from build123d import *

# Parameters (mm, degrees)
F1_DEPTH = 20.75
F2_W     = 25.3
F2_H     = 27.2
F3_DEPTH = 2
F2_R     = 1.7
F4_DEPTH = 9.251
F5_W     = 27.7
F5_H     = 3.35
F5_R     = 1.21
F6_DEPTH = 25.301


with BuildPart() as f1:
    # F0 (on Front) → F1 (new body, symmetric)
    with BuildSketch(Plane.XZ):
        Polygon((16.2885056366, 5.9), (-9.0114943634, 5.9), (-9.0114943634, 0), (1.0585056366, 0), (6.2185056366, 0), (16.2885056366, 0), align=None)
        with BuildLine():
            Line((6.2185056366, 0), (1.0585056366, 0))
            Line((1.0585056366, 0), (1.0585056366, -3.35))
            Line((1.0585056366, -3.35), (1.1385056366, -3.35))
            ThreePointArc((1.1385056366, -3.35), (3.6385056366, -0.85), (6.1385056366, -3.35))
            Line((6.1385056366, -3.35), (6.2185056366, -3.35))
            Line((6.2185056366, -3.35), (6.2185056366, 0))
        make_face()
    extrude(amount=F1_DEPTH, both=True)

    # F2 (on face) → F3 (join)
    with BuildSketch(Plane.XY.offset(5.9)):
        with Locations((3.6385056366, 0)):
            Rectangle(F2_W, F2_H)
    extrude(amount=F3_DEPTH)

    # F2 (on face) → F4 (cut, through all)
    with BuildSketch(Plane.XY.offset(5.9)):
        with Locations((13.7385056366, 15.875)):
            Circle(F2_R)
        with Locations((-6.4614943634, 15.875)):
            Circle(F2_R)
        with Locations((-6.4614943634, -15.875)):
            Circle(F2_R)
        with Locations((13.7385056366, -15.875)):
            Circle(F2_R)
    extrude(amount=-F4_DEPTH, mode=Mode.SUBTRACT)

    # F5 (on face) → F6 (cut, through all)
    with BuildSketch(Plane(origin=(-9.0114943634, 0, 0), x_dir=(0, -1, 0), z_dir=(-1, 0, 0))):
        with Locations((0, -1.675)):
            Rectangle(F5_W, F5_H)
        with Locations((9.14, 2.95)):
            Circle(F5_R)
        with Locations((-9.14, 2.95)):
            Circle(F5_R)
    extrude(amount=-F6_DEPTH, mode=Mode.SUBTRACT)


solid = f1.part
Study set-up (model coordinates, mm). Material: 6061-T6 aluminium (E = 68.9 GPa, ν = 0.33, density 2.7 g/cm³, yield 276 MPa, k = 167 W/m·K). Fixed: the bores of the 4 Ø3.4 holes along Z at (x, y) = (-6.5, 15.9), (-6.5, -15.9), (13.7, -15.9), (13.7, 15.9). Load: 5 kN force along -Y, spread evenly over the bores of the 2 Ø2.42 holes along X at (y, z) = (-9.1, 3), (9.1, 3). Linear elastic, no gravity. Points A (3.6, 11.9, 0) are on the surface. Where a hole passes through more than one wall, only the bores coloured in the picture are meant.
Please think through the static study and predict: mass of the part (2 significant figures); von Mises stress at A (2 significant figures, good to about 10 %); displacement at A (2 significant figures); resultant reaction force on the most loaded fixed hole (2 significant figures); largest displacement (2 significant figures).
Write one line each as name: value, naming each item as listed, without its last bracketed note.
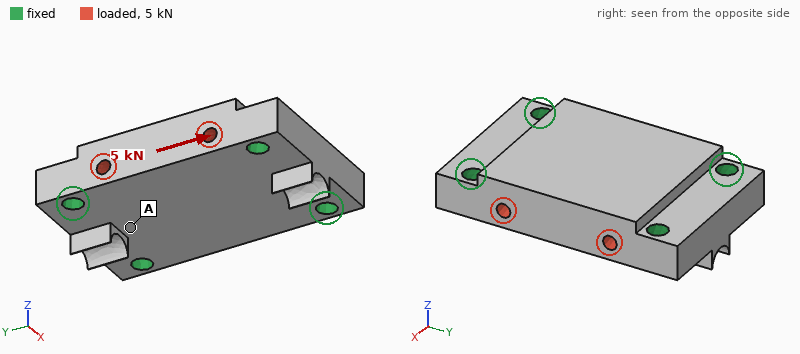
mass of the part: 20 g
von Mises stress at A: 7.4 MPa
displacement at A: 3.0 µm
resultant reaction force on the most loaded fixed hole: 1.3 kN
largest displacement: 3.5 µm
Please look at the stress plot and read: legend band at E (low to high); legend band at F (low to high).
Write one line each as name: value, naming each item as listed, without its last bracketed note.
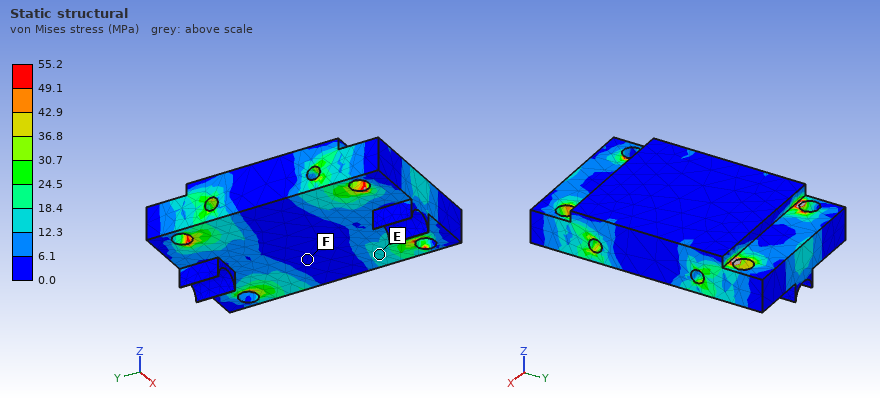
legend band at E: 12.3 to 18.4 MPa
legend band at F: 0.0 to 6.1 MPa
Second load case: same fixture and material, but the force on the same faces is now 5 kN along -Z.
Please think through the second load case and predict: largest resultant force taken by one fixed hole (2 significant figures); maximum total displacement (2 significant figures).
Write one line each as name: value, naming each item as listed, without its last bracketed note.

largest resultant force taken by one fixed hole: 1.3 kN
maximum total displacement: 15 µm
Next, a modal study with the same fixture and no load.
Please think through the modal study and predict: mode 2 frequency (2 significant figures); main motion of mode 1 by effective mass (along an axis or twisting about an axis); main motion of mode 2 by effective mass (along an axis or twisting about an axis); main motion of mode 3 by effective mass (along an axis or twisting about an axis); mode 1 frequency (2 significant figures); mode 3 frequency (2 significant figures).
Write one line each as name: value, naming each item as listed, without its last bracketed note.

mode 2 frequency: 33 kHz
main motion of mode 1 by effective mass: along Z
main motion of mode 2 by effective mass: twisting about Y
main motion of mode 3 by effective mass: along X
mode 1 frequency: 24 kHz
mode 3 frequency: 39 kHz
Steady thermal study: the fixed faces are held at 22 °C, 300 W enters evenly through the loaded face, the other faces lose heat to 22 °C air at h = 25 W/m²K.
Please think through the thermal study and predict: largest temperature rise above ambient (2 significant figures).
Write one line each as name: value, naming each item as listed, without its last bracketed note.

largest temperature rise above ambient: 51 K
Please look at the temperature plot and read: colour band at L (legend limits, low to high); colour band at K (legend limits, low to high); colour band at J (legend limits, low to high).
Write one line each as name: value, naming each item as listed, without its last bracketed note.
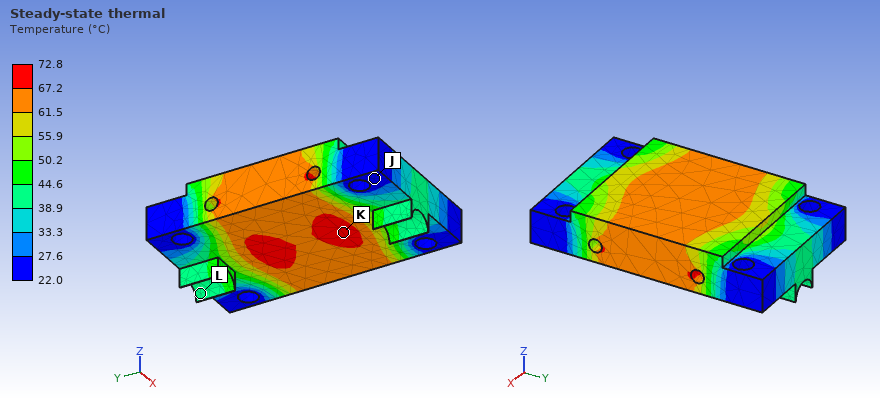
colour band at L: 38.9 to 44.6 °C
colour band at K: 67.2 to 72.8 °C
colour band at J: 22.0 to 27.6 °C
